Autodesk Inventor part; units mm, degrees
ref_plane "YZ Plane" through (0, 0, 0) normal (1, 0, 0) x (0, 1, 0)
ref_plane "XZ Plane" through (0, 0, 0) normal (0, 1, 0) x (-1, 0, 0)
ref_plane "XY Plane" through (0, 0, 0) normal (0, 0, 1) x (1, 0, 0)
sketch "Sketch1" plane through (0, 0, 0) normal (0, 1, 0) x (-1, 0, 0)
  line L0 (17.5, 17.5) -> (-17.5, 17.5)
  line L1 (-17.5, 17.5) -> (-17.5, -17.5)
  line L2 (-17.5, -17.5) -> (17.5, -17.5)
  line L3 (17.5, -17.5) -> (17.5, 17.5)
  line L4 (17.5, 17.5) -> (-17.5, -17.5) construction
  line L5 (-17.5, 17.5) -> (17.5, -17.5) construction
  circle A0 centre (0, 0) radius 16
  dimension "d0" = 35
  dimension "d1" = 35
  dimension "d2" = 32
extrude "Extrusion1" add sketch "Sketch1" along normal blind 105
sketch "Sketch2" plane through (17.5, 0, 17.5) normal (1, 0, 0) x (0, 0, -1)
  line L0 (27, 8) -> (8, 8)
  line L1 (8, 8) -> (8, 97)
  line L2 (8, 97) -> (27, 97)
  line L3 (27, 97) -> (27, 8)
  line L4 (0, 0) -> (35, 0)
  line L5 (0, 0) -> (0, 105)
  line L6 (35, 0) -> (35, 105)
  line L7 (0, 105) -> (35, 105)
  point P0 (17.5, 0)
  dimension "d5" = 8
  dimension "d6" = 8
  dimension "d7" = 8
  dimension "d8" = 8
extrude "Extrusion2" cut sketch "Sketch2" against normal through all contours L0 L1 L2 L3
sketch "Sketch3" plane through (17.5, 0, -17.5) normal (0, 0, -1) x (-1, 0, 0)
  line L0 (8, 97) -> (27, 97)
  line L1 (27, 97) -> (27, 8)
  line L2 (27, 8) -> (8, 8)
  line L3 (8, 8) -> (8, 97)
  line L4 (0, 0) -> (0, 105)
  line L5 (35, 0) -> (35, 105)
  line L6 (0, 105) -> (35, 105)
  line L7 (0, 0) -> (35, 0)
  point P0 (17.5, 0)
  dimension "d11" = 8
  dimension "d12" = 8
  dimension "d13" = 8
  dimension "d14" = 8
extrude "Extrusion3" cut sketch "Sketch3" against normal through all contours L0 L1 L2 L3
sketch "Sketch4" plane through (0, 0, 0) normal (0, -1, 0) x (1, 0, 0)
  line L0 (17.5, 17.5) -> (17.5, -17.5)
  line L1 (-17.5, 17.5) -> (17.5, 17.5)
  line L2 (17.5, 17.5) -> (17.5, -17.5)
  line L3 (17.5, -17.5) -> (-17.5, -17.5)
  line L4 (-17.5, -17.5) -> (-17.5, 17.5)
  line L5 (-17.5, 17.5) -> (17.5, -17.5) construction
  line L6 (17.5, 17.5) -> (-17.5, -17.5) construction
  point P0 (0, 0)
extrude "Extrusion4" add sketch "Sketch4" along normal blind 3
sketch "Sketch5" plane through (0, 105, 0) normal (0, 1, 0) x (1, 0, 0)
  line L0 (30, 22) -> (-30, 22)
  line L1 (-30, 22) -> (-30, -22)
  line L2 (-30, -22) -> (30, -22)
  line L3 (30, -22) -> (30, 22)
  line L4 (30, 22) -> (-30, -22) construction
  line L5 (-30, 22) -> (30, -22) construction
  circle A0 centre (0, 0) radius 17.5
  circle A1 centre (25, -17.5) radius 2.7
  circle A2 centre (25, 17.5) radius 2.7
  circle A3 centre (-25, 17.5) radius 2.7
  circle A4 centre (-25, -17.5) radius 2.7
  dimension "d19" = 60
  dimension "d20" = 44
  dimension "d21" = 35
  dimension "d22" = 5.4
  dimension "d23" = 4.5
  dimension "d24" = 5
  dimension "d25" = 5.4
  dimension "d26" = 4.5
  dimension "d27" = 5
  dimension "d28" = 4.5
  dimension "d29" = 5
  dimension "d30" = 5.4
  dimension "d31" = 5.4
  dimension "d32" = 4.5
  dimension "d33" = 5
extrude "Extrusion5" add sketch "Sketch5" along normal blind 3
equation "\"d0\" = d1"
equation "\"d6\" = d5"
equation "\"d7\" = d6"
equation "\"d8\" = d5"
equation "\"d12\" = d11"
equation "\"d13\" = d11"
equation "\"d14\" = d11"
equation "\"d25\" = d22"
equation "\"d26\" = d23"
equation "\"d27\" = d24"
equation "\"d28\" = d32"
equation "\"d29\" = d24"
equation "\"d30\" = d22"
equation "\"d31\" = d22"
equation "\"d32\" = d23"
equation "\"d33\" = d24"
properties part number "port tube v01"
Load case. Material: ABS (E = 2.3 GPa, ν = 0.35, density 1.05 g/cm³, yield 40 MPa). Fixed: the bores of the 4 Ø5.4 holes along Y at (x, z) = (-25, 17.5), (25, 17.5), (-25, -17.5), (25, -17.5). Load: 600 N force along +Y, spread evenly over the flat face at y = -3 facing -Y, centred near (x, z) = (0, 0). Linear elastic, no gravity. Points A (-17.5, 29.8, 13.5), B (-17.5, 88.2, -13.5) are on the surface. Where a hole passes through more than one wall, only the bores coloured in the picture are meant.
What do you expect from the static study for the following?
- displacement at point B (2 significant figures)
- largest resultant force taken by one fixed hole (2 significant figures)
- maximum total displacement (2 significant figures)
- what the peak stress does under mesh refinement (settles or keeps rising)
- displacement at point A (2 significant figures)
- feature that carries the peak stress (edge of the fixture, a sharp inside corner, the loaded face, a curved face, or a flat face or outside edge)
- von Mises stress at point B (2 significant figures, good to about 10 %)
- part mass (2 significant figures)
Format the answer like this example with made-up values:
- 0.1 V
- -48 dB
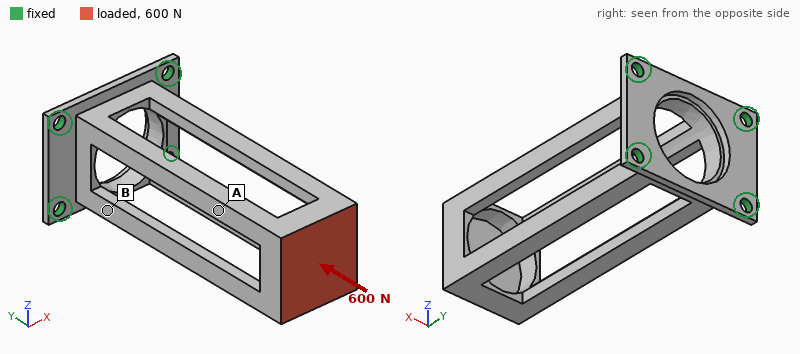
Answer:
- 0.20 mm
- 170 N
- 0.48 mm
- keeps rising
- 0.27 mm
- edge of the fixture
- 4.6 MPa
- 38 g
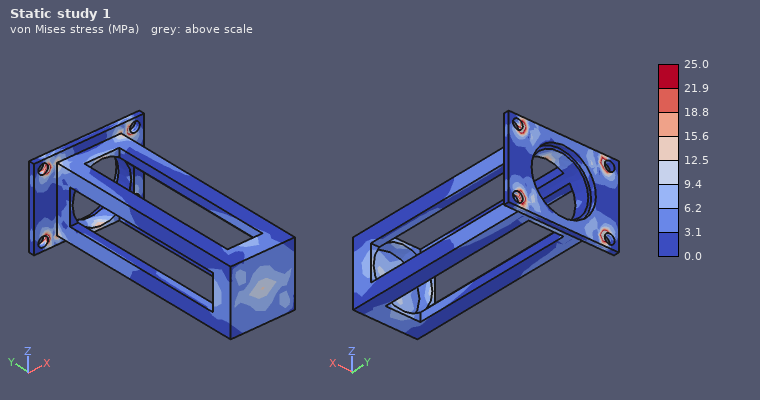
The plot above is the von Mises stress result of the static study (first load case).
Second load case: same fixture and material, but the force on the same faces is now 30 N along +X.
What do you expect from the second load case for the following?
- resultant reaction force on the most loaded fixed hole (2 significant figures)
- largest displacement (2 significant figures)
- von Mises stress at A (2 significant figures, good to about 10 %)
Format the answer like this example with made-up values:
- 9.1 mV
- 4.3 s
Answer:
- 42 N
- 1.3 mm
- 1.6 MPa
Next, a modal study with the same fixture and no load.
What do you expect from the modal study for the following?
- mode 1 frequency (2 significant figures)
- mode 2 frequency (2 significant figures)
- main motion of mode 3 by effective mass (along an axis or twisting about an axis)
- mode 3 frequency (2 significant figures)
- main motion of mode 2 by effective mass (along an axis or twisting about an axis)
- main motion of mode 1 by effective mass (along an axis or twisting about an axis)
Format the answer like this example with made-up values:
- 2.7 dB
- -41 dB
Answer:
- 190 Hz
- 200 Hz
- twisting about Y
- 390 Hz
- along X
- along Z
